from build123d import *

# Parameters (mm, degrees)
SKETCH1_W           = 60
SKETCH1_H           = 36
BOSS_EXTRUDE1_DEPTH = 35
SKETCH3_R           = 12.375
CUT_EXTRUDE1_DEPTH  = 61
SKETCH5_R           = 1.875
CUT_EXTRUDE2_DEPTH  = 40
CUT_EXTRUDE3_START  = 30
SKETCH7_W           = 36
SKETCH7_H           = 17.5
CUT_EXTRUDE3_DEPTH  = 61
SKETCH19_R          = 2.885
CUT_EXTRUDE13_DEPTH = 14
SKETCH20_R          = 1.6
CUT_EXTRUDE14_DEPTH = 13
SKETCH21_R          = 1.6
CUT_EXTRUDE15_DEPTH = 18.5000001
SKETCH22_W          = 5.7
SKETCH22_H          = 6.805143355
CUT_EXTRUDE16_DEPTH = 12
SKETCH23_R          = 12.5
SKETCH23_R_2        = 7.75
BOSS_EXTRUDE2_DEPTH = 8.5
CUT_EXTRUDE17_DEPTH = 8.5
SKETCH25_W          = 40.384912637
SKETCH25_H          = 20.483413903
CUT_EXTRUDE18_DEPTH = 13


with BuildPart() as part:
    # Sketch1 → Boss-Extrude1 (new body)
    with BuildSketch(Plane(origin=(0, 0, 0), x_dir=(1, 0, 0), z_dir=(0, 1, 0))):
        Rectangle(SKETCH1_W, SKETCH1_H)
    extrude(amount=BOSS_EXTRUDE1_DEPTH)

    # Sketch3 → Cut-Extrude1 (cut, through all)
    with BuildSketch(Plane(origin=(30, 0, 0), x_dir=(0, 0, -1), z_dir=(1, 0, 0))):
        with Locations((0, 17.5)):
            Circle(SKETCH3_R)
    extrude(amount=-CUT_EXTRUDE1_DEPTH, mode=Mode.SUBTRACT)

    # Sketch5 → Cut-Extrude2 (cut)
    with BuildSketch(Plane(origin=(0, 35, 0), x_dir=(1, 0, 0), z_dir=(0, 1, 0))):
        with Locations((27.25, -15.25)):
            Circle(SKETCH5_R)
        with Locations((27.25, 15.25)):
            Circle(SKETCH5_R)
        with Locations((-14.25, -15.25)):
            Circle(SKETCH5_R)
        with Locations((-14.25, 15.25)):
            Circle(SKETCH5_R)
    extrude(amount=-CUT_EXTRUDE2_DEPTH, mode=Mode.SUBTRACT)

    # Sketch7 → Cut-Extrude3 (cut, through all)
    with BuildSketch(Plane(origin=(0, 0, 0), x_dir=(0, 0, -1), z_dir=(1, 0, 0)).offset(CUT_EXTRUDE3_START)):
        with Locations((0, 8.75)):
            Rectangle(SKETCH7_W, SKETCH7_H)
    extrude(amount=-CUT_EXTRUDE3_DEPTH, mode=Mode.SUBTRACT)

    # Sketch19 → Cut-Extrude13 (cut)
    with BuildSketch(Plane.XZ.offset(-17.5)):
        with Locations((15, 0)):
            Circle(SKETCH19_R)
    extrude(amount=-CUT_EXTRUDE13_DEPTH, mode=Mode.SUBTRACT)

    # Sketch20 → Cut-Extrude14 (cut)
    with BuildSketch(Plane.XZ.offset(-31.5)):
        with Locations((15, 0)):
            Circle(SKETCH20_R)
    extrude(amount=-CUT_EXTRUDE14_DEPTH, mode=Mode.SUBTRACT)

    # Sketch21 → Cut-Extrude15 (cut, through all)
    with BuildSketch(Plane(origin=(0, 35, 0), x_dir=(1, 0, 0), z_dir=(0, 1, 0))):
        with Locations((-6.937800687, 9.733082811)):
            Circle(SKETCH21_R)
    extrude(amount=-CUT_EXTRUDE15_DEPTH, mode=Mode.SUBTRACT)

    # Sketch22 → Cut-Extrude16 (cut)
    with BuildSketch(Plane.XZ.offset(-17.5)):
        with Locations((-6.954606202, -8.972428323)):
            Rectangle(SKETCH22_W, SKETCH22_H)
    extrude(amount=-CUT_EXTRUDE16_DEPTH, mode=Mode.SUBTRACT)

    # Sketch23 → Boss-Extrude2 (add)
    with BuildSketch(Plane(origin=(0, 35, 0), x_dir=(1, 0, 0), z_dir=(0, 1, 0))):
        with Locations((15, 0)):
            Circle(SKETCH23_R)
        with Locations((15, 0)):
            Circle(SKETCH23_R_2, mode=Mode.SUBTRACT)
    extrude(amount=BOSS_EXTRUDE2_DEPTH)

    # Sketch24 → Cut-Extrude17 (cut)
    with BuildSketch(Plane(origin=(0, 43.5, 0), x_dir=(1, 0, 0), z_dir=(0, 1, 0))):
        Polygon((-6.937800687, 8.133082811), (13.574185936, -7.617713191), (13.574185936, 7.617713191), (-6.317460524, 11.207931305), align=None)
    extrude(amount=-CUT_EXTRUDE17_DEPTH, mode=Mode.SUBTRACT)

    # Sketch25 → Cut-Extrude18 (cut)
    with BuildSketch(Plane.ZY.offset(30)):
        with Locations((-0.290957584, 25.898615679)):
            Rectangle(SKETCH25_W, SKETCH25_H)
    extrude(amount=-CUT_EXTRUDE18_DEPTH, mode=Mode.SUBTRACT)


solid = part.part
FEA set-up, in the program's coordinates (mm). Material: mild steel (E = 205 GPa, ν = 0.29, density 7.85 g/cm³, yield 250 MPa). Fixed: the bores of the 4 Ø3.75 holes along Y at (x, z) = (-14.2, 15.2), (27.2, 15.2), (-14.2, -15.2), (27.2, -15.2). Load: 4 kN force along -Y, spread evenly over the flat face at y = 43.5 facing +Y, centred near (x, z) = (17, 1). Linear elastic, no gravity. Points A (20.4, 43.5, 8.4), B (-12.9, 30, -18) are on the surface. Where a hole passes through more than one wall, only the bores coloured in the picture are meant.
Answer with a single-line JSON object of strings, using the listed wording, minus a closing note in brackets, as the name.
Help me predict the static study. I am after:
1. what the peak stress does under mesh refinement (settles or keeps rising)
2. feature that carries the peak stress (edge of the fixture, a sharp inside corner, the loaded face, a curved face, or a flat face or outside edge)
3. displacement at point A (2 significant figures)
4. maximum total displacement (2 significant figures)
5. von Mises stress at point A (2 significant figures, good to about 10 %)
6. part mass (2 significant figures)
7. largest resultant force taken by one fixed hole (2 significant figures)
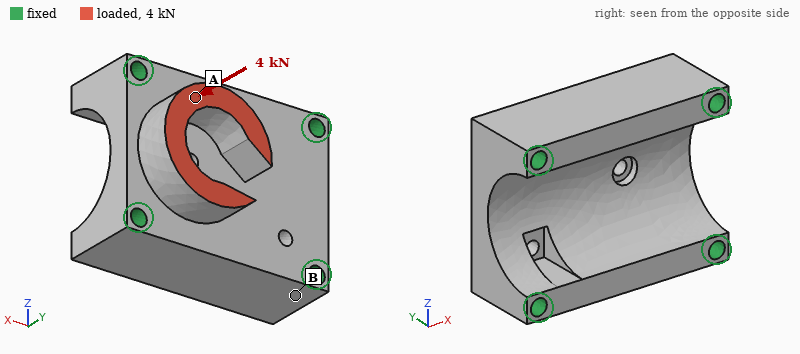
{"what the peak stress does under mesh refinement": "keeps rising", "feature that carries the peak stress": "edge of the fixture", "displacement at point A": "2.4 µm", "maximum total displacement": "3.7 µm", "von Mises stress at point A": "17 MPa", "part mass": "150 g", "largest resultant force taken by one fixed hole": "1.8 kN"}
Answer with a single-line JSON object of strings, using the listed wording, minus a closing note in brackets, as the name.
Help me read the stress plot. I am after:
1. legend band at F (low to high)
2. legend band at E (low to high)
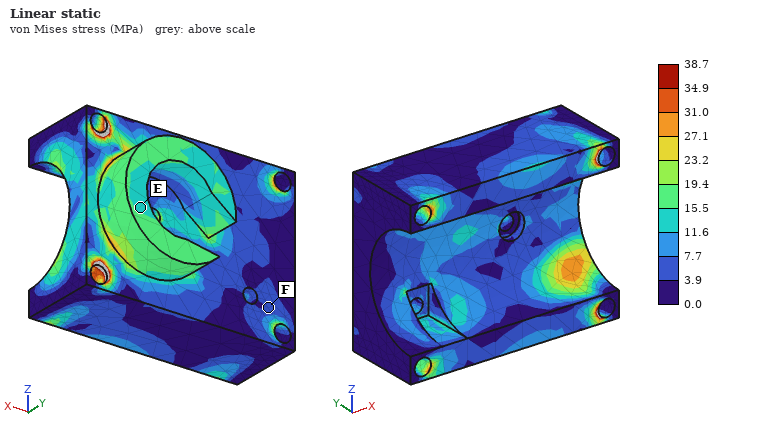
{"legend band at F": "3.9 to 7.7 MPa", "legend band at E": "11.6 to 15.5 MPa"}
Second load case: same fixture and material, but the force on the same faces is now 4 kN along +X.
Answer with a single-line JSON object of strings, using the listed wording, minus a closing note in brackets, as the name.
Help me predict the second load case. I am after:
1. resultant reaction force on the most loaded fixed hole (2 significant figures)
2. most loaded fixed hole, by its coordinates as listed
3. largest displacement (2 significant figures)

{"resultant reaction force on the most loaded fixed hole": "1.6 kN", "most loaded fixed hole, by its coordinates as listed": "(27.2, 15.2)", "largest displacement": "13 µm"}
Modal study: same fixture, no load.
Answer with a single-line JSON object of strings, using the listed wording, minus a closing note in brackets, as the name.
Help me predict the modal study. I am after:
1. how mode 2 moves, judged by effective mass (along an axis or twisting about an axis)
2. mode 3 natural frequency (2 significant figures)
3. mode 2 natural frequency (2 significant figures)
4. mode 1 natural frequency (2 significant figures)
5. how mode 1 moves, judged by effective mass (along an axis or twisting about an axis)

{"how mode 2 moves, judged by effective mass": "along Z", "mode 3 natural frequency": "28 kHz", "mode 2 natural frequency": "25 kHz", "mode 1 natural frequency": "22 kHz", "how mode 1 moves, judged by effective mass": "along Y"}
